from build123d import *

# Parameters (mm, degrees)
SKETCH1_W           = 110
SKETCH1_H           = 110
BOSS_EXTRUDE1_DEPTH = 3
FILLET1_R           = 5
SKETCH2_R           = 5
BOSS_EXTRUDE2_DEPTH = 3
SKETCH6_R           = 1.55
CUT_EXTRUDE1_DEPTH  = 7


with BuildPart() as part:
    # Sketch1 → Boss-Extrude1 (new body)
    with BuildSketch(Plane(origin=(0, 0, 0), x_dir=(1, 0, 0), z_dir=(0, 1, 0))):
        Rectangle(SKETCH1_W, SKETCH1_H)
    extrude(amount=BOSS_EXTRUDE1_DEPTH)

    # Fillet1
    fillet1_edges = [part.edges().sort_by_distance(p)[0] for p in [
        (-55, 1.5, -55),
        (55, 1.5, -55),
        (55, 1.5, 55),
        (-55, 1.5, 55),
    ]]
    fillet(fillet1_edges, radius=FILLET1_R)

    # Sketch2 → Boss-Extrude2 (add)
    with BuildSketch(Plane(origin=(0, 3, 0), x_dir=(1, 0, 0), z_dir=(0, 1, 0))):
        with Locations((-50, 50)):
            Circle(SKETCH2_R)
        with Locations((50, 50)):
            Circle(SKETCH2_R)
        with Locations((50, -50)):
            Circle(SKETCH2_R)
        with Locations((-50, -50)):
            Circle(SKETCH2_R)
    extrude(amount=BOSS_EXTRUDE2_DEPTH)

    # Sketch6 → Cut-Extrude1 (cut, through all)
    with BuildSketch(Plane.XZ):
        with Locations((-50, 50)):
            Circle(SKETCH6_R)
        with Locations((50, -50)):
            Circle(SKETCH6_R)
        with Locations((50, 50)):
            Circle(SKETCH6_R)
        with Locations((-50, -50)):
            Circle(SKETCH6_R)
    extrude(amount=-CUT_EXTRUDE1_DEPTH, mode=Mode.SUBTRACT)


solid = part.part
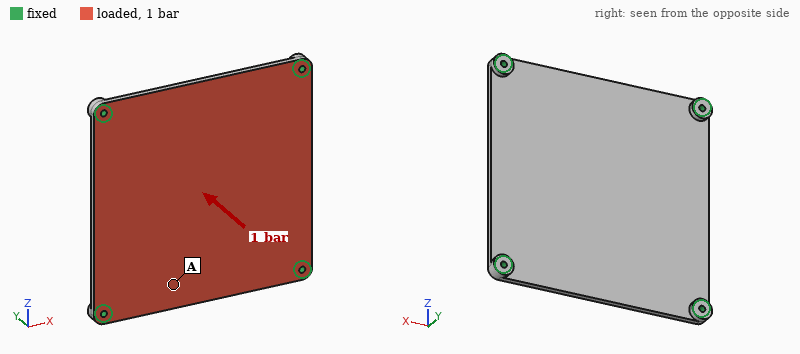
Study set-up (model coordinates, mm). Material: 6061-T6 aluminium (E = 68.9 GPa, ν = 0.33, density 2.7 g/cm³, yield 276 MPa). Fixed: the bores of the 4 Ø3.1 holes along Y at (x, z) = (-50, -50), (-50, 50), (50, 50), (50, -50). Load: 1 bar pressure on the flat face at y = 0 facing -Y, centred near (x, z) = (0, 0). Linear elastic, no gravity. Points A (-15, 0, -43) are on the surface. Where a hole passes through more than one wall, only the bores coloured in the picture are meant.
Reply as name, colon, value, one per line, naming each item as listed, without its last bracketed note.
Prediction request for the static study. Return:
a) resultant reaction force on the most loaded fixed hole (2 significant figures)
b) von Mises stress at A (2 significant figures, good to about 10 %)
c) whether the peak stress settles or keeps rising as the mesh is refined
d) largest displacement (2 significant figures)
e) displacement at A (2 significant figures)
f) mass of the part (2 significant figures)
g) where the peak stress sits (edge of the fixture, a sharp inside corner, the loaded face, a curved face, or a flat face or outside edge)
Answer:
resultant reaction force on the most loaded fixed hole: 350 N
von Mises stress at A: 30 MPa
whether the peak stress settles or keeps rising as the mesh is refined: keeps rising
largest displacement: 0.44 mm
displacement at A: 0.23 mm
mass of the part: 100 g
where the peak stress sits: edge of the fixture
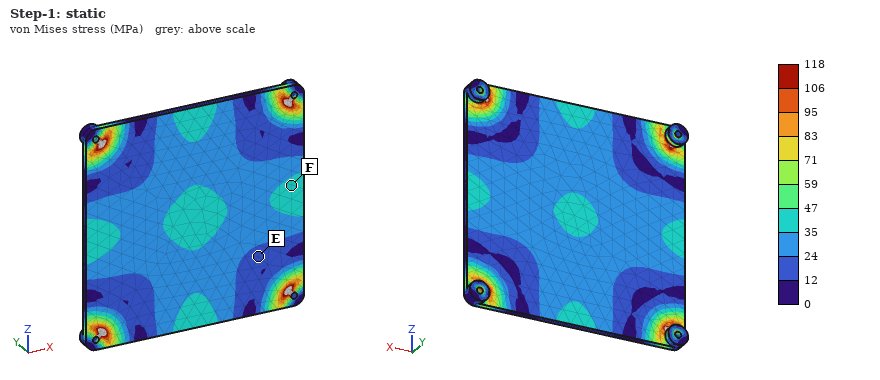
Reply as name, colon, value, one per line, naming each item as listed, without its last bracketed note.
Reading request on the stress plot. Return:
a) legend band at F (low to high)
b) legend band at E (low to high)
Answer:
legend band at F: 35 to 47 MPa
legend band at E: 12 to 24 MPa
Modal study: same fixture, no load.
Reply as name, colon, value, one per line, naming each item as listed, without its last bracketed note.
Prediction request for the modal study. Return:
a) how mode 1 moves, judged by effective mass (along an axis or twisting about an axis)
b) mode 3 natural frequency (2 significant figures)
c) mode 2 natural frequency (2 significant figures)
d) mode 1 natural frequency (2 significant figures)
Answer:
how mode 1 moves, judged by effective mass: along Y
mode 3 natural frequency: 1800 Hz
mode 2 natural frequency: 1800 Hz
mode 1 natural frequency: 1000 Hz
